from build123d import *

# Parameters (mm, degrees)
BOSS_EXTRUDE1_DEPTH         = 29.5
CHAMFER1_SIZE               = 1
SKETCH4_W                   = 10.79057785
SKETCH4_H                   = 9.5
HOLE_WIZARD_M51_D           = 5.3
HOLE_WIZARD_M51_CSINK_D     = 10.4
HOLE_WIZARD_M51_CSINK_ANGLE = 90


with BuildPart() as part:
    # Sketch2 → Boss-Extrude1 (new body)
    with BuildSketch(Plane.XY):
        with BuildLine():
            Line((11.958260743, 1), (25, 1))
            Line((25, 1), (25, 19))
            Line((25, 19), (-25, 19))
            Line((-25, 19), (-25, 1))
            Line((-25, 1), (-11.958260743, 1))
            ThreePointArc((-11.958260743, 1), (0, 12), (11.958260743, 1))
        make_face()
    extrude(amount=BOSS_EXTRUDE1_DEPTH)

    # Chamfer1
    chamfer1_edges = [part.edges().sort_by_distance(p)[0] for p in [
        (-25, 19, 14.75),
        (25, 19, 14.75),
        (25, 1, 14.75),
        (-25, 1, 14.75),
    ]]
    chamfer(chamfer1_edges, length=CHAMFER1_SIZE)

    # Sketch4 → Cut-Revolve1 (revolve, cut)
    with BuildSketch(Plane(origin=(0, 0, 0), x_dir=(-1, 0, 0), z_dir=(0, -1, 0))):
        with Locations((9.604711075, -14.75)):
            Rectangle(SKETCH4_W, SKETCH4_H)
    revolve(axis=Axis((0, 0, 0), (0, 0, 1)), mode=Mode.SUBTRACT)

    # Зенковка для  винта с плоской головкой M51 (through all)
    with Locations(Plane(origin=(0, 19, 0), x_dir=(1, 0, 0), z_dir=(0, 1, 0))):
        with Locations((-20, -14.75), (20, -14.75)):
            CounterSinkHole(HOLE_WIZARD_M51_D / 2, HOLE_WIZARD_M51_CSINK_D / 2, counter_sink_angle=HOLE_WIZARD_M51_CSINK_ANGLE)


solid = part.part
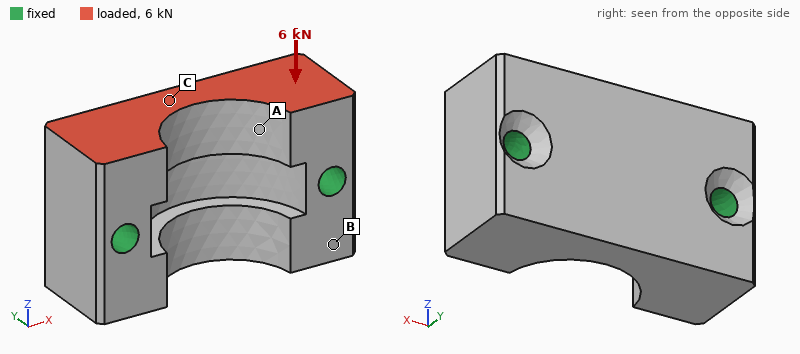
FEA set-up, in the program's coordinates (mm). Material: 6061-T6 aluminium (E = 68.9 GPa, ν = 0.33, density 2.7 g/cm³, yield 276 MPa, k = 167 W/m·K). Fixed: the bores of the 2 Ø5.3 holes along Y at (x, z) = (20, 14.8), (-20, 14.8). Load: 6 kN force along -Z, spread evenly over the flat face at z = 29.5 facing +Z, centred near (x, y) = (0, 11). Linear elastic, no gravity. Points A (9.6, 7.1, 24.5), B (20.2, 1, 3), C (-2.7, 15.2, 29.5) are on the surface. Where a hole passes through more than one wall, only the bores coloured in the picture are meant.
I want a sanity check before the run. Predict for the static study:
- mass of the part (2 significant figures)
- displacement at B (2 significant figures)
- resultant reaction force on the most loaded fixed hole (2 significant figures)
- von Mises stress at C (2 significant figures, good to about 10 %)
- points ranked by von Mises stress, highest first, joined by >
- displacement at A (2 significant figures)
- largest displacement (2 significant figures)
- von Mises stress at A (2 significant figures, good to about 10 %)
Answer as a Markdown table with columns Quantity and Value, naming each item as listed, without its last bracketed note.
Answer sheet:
| Quantity | Value |
|---|---|
| mass of the part | 50 g |
| displacement at B | 1.5 µm |
| resultant reaction force on the most loaded fixed hole | 3.0 kN |
| von Mises stress at C | 12 MPa |
| points ranked by von Mises stress, highest first, joined by > | C > A > B |
| displacement at A | 4.0 µm |
| largest displacement | 6.7 µm |
| von Mises stress at A | 6.0 MPa |
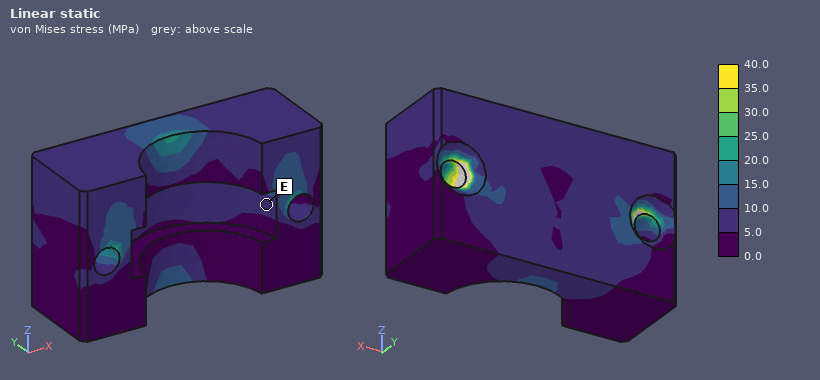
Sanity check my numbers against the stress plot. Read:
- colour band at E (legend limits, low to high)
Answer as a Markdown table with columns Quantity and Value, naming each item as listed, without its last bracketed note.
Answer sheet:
| Quantity | Value |
|---|---|
| colour band at E | 5.0 to 10.0 MPa |
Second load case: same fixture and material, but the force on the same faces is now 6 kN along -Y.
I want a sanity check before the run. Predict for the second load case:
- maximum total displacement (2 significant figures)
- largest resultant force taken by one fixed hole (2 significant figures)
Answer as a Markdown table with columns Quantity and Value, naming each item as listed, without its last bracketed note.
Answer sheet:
| Quantity | Value |
|---|---|
| maximum total displacement | 27 µm |
| largest resultant force taken by one fixed hole | 3.1 kN |
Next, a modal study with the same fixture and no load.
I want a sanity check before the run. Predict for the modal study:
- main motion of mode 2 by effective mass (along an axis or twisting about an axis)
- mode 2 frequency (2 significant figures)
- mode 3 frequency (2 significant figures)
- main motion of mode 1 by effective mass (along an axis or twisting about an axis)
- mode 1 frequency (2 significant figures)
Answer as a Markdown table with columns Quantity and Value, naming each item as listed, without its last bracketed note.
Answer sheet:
| Quantity | Value |
|---|---|
| main motion of mode 2 by effective mass | along Y |
| mode 2 frequency | 26 kHz |
| mode 3 frequency | 32 kHz |
| main motion of mode 1 by effective mass | along Z |
| mode 1 frequency | 24 kHz |
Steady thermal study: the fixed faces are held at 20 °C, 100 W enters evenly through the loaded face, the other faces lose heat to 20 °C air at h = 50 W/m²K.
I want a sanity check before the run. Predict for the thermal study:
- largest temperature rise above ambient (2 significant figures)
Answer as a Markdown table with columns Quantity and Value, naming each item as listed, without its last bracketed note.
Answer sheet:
| Quantity | Value |
|---|---|
| largest temperature rise above ambient | 17 K |
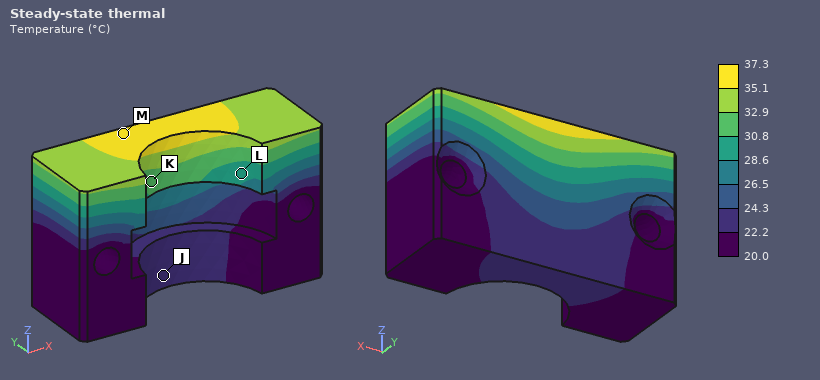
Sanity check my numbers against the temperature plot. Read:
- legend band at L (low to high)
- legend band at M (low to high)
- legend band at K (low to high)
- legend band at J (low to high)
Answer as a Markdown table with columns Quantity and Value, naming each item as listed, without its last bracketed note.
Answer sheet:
| Quantity | Value |
|---|---|
| legend band at L | 28.6 to 30.8 °C |
| legend band at M | 35.1 to 37.3 °C |
| legend band at K | 30.8 to 32.9 °C |
| legend band at J | 22.2 to 24.3 °C |
